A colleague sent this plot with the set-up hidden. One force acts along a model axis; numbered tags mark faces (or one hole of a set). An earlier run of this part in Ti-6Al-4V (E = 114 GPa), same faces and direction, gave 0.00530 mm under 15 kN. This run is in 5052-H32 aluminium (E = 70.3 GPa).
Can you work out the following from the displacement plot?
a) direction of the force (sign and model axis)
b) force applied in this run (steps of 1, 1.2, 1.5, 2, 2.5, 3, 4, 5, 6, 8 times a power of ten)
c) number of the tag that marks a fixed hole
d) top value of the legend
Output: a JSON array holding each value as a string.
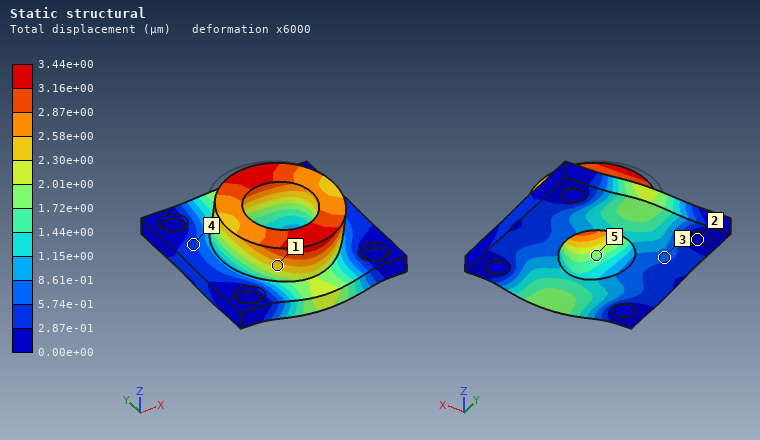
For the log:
["-Y", "6 kN", "2", "3.44e+00 µm"]
